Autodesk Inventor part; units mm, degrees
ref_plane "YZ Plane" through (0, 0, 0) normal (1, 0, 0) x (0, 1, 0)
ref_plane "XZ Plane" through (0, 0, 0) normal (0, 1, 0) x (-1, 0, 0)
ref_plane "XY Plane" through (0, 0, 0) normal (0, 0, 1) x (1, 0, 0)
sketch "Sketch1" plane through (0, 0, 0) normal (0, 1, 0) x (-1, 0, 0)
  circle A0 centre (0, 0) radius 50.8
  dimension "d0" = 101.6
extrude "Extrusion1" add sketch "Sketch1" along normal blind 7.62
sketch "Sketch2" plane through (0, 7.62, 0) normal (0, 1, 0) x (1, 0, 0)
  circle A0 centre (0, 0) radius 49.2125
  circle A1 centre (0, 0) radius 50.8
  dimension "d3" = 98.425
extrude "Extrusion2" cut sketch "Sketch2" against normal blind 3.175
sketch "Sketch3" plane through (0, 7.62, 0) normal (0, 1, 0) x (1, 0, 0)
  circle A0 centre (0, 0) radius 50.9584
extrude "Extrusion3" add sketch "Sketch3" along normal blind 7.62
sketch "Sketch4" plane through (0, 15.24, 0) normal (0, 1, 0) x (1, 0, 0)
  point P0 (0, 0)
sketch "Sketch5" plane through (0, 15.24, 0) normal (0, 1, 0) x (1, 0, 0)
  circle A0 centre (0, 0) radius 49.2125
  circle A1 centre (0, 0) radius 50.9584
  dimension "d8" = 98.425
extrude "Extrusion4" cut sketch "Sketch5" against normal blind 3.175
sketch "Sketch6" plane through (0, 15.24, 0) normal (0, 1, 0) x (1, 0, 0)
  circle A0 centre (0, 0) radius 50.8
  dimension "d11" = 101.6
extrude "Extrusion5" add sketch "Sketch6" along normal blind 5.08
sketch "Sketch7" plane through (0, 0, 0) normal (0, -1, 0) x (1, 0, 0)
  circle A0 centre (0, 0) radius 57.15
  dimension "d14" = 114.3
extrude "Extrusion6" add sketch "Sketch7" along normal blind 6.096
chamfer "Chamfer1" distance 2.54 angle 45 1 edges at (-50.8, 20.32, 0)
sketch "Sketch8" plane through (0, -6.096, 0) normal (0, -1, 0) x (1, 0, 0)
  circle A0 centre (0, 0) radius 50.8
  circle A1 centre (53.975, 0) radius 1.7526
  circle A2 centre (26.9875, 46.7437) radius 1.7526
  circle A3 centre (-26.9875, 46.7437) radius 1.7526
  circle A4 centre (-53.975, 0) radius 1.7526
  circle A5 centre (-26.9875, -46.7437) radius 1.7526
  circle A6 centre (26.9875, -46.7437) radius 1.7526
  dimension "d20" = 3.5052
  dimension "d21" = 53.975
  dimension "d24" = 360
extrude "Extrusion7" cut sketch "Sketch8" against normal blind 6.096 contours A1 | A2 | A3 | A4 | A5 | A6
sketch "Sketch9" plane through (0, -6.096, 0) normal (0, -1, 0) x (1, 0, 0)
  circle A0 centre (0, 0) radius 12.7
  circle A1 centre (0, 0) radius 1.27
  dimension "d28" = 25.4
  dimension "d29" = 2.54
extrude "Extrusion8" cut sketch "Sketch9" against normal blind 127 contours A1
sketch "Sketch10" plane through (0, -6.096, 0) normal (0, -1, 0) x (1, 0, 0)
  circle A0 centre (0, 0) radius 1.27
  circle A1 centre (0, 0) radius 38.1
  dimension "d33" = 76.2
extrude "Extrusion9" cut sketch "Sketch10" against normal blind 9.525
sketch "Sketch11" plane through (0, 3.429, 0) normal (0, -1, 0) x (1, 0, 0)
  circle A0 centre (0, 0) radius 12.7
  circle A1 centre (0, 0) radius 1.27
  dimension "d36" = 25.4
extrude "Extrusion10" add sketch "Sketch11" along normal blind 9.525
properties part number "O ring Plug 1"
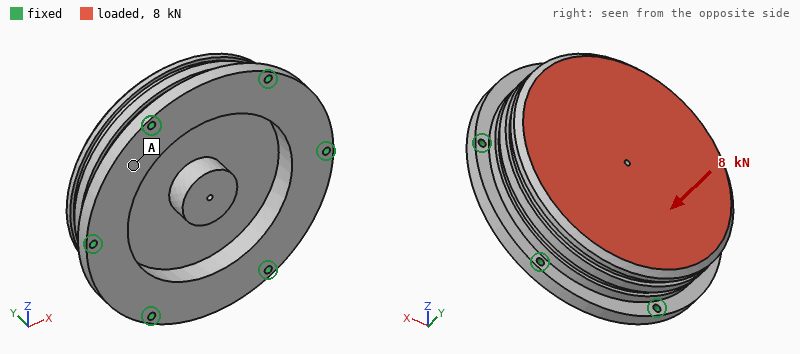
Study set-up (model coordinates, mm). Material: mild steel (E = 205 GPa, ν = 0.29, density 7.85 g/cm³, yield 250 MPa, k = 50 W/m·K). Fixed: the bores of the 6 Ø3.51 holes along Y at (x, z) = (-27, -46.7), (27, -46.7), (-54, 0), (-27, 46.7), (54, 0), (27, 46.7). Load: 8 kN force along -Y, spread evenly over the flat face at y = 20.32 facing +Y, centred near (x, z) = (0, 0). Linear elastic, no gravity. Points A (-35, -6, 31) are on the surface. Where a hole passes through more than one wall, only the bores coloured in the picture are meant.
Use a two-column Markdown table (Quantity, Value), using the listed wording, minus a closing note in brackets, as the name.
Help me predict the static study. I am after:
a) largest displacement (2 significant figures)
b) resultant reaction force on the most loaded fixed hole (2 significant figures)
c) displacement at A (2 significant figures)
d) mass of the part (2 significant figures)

| Quantity | Value |
|---|---|
| largest displacement | 4.0 µm |
| resultant reaction force on the most loaded fixed hole | 1.6 kN |
| displacement at A | 2.3 µm |
| mass of the part | 1.4 kg |
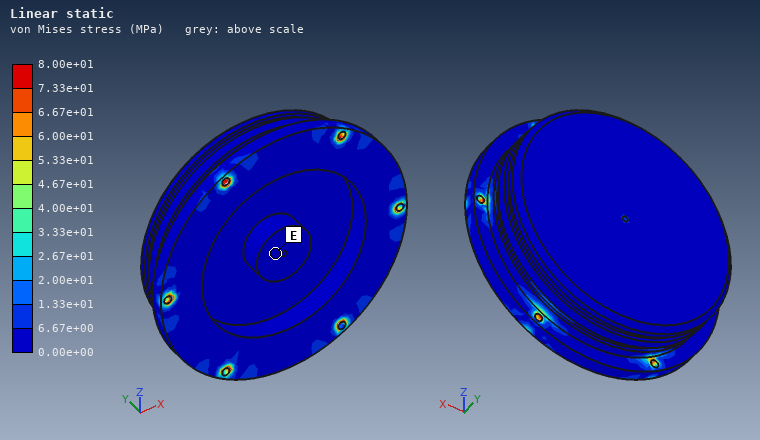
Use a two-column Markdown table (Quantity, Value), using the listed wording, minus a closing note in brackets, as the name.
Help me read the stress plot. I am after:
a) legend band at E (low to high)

| Quantity | Value |
|---|---|
| legend band at E | 0.00e+00 to 6.67e+00 MPa |
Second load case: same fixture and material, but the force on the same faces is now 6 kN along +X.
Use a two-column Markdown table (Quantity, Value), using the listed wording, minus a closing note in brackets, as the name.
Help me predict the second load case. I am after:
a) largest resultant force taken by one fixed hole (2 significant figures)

| Quantity | Value |
|---|---|
| largest resultant force taken by one fixed hole | 1.4 kN |
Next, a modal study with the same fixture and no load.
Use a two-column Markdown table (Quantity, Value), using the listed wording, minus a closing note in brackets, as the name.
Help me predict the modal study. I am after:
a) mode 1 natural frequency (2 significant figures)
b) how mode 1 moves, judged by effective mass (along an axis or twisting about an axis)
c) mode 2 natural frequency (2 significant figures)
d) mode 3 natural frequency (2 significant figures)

| Quantity | Value |
|---|---|
| mode 1 natural frequency | 7300 Hz |
| how mode 1 moves, judged by effective mass | along Y |
| mode 2 natural frequency | 9500 Hz |
| mode 3 natural frequency | 9600 Hz |
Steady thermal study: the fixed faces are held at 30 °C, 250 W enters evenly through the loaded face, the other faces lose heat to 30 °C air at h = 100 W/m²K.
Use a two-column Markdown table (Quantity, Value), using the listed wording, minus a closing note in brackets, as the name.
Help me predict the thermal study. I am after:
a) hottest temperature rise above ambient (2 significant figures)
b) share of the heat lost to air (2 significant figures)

| Quantity | Value |
|---|---|
| hottest temperature rise above ambient | 65 K |
| share of the heat lost to air | 42 % |
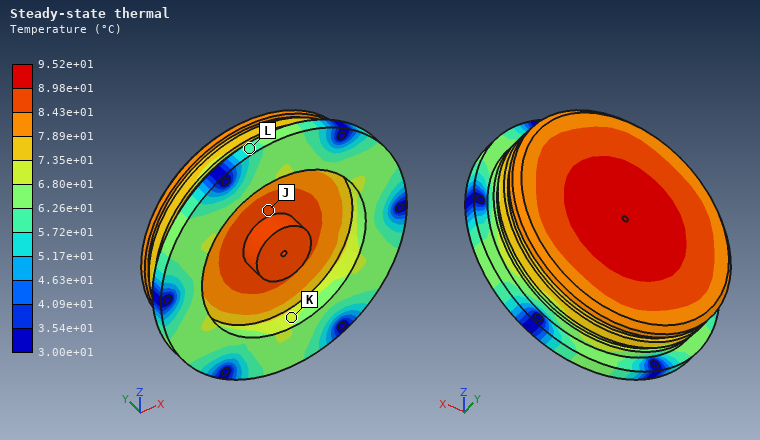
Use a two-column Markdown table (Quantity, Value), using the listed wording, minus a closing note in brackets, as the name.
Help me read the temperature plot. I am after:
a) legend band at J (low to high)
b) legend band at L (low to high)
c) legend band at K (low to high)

| Quantity | Value |
|---|---|
| legend band at J | 8.43e+01 to 8.98e+01 °C |
| legend band at L | 5.72e+01 to 6.26e+01 °C |
| legend band at K | 6.80e+01 to 7.35e+01 °C |
